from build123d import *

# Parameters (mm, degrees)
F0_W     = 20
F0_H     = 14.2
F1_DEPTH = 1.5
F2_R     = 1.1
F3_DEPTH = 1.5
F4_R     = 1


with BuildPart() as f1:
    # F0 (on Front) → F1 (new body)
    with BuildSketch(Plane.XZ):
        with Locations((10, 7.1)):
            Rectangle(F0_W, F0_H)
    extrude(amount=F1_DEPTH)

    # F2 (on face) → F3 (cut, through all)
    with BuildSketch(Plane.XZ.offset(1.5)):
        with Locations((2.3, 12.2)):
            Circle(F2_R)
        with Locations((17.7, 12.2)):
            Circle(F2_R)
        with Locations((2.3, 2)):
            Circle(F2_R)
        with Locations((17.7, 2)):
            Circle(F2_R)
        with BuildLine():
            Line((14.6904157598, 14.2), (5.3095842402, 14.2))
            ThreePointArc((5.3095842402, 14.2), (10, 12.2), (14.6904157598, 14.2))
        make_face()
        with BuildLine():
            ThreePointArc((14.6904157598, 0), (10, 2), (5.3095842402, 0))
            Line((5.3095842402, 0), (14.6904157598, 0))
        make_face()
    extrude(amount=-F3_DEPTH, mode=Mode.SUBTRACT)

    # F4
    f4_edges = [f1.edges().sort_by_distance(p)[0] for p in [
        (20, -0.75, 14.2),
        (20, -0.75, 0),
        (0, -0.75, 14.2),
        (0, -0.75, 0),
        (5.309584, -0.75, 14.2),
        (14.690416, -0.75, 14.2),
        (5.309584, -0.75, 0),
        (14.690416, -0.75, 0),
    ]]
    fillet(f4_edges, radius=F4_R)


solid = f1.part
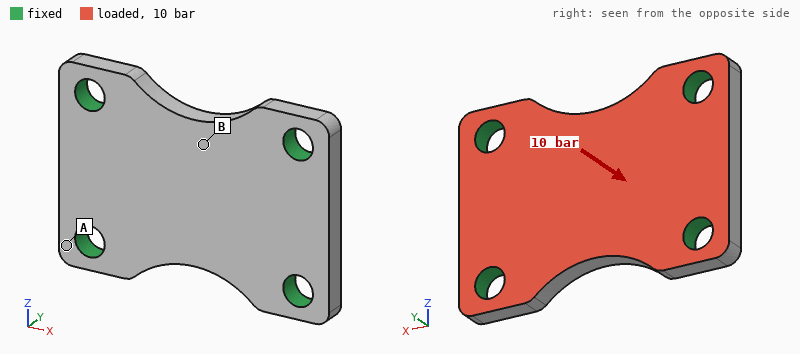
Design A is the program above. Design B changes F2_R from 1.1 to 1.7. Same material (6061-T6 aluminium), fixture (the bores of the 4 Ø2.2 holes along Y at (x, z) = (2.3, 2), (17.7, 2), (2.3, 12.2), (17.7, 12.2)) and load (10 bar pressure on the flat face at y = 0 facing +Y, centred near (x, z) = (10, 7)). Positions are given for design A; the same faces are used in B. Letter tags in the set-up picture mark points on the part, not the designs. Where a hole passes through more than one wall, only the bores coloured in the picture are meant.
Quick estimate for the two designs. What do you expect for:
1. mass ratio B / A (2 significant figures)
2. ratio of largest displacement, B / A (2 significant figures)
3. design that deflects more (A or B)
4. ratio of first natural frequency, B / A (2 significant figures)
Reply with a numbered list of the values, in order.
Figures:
1. 0.91
2. 0.69
3. A
4. 1.2
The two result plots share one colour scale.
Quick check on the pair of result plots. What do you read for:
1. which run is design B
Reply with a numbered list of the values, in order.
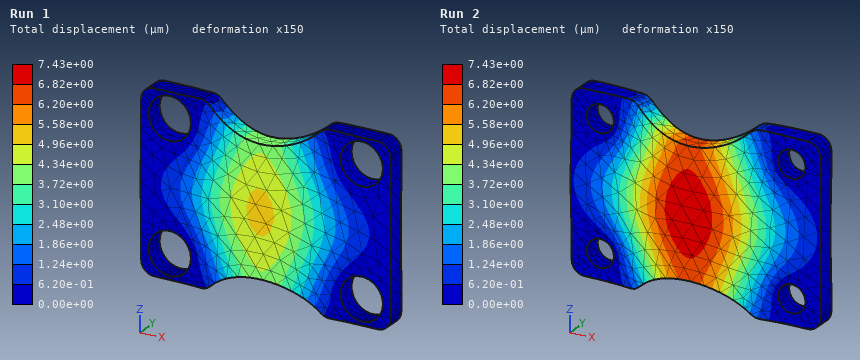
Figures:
1. Run 1
